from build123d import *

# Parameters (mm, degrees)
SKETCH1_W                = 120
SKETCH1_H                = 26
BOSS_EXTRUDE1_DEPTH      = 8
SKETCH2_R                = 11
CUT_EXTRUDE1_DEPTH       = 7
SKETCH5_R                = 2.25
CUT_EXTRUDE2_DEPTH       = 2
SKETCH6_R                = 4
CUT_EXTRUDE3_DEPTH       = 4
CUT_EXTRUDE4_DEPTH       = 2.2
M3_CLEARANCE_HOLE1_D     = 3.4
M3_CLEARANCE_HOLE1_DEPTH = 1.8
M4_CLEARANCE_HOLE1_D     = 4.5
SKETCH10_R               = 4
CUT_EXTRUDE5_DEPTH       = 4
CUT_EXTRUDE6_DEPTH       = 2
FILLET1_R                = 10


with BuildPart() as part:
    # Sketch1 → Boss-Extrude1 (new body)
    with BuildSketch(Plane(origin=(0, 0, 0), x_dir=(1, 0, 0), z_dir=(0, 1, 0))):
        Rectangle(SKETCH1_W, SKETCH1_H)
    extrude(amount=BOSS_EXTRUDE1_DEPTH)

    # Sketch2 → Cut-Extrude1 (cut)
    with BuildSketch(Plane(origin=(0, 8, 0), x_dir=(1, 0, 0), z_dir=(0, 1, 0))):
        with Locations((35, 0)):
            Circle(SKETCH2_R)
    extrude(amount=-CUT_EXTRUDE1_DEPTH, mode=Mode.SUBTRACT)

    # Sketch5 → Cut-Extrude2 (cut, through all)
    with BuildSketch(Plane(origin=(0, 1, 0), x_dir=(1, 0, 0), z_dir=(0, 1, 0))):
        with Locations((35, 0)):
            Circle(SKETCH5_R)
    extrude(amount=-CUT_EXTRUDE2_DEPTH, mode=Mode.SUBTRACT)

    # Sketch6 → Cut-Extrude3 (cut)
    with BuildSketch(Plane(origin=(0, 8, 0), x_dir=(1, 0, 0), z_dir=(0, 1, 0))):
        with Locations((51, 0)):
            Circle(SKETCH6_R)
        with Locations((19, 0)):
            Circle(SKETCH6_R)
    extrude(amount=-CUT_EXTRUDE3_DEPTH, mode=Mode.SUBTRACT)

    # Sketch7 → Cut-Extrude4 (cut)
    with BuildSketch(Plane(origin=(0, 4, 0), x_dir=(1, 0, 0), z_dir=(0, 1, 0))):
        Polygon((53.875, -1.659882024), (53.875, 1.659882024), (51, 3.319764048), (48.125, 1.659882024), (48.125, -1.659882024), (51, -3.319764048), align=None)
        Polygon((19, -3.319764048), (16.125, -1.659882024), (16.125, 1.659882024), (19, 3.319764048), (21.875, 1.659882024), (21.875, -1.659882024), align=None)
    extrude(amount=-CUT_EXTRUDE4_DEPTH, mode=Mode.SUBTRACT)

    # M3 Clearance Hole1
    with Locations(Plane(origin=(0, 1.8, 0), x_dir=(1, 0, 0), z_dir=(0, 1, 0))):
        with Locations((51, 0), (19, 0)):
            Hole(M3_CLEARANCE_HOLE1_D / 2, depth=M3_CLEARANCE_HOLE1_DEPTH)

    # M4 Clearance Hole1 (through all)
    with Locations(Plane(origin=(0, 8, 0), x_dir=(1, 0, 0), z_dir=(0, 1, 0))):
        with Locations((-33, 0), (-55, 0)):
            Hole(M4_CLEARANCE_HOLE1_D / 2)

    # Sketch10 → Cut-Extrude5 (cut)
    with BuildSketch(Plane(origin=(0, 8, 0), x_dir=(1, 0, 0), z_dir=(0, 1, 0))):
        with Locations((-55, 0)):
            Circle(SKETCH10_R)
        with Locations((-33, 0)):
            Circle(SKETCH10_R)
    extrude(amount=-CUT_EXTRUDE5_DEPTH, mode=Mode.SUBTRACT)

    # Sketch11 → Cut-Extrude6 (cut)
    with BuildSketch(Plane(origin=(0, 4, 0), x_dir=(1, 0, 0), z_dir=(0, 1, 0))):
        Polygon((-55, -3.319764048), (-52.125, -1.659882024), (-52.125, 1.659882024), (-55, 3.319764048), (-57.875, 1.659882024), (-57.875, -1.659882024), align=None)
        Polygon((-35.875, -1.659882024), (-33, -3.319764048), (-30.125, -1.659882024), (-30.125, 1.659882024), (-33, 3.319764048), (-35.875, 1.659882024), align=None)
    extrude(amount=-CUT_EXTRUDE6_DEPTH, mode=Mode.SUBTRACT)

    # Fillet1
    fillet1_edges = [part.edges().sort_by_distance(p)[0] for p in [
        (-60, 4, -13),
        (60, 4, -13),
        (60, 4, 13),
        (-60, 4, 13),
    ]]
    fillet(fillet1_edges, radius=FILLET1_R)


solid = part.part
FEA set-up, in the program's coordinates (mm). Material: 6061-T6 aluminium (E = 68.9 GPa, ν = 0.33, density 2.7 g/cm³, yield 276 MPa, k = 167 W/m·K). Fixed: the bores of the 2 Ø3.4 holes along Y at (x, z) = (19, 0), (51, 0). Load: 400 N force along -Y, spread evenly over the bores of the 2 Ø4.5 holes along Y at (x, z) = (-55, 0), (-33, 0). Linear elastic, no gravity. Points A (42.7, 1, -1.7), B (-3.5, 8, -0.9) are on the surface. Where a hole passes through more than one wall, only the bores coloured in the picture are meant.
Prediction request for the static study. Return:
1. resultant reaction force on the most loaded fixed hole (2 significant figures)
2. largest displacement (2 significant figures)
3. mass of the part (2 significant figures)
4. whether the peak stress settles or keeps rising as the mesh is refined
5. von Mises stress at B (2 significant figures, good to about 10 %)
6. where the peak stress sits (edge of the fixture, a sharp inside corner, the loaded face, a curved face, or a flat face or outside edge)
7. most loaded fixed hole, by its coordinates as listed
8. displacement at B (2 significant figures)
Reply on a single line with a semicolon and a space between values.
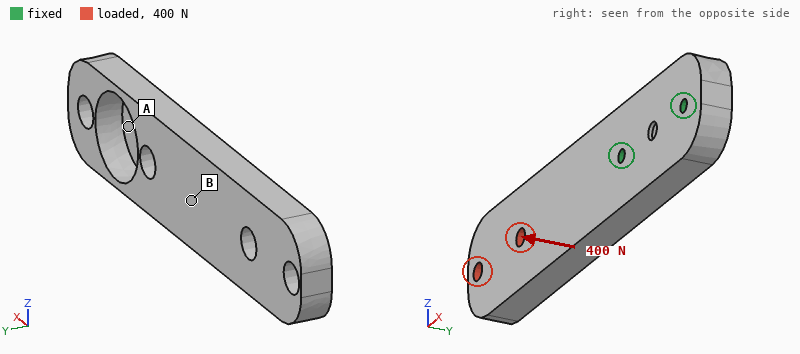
1.5 kN; 1.1 mm; 55 g; keeps rising; 55 MPa; edge of the fixture; (19, 0); 0.22 mm
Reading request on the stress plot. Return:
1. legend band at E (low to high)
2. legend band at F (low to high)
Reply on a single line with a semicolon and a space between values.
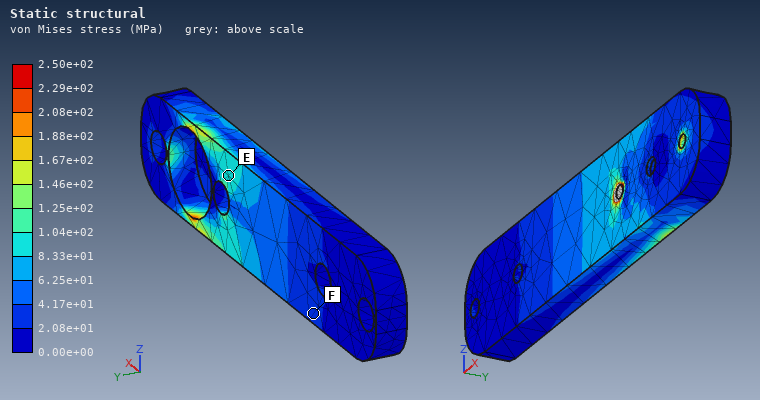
8.33e+01 to 1.04e+02 MPa; 2.08e+01 to 4.17e+01 MPa
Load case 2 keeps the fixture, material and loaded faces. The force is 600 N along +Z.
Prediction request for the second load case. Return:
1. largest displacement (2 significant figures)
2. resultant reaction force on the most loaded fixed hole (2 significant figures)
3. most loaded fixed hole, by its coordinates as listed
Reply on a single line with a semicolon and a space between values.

0.28 mm; 1.6 kN; (19, 0)
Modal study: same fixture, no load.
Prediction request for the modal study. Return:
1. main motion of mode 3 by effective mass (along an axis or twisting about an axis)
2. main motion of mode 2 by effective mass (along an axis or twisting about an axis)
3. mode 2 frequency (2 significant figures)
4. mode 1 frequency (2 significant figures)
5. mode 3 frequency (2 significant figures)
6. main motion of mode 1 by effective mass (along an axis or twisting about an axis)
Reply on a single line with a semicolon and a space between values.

twisting about X; along Z; 1900 Hz; 810 Hz; 2800 Hz; along Y
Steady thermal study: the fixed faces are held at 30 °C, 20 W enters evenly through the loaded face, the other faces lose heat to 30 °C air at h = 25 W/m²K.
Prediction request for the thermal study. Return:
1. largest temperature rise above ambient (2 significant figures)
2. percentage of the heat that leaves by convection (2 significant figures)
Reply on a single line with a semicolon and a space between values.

45 K; 20 %
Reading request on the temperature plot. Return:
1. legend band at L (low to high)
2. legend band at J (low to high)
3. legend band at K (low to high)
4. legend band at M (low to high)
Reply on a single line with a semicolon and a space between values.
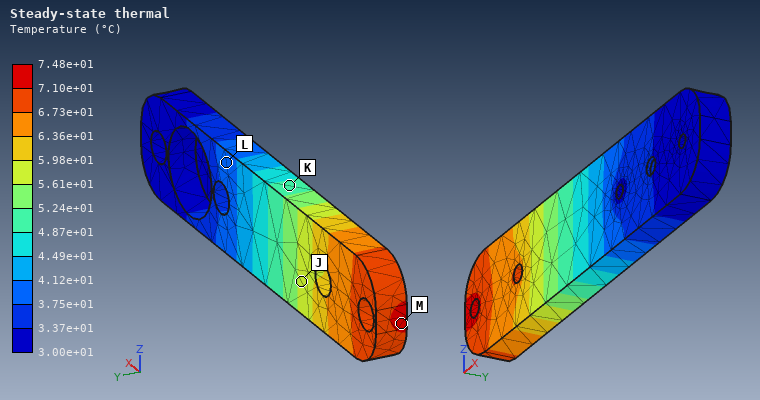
3.75e+01 to 4.12e+01 °C; 5.61e+01 to 5.98e+01 °C; 4.87e+01 to 5.24e+01 °C; 7.10e+01 to 7.48e+01 °C
